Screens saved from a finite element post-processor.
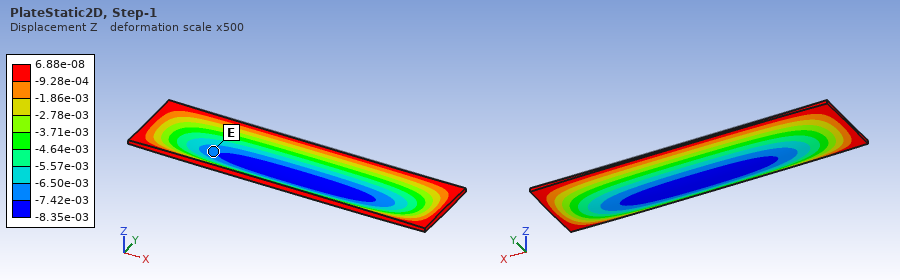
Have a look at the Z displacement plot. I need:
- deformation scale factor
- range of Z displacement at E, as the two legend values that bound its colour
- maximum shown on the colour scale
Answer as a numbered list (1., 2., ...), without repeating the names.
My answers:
1. 500
2. -7.42e-03 to -6.50e-03
3. 6.88e-08
